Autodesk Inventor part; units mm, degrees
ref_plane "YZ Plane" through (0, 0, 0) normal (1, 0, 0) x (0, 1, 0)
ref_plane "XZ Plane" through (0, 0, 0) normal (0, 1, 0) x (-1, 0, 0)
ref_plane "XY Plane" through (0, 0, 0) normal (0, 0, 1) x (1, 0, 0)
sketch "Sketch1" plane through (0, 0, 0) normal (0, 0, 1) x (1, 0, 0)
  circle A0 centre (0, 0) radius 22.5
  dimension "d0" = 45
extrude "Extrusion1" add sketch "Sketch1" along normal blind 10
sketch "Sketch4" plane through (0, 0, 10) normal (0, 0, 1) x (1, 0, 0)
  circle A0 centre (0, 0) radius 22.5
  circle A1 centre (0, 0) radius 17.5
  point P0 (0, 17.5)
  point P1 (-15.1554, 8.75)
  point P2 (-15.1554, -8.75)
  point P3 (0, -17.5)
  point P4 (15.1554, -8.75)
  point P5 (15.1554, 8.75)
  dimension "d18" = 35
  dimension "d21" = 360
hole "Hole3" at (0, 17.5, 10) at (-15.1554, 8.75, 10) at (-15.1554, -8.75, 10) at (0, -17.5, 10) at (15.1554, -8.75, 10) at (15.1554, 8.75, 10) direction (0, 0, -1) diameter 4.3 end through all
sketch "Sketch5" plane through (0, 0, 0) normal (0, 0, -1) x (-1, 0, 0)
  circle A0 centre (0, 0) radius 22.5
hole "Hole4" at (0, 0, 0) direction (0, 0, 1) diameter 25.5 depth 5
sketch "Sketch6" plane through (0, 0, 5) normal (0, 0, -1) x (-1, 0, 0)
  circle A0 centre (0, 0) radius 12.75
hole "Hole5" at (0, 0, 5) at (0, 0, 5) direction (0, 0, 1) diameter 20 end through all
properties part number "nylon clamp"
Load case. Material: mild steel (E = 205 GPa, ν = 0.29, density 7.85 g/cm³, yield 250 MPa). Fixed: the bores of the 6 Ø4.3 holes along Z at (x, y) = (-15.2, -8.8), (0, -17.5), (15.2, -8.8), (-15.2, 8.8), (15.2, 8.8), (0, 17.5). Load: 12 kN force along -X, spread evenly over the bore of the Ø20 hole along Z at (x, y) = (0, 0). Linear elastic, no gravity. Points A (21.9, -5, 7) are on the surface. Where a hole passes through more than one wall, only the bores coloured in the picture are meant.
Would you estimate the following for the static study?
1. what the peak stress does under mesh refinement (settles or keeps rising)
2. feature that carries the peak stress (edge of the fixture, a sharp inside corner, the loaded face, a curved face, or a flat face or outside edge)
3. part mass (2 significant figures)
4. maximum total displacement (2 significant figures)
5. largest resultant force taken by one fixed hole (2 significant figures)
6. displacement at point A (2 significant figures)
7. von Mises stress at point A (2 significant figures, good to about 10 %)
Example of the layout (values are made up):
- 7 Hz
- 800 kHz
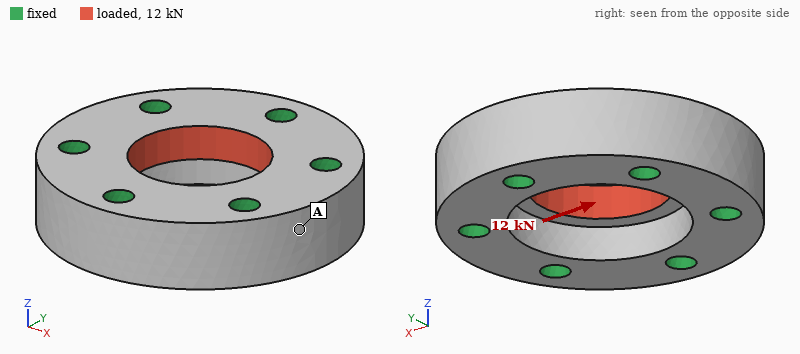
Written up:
- keeps rising
- edge of the fixture
- 86 g
- 2.3 µm
- 2.4 kN
- 0.61 µm
- 11 MPa
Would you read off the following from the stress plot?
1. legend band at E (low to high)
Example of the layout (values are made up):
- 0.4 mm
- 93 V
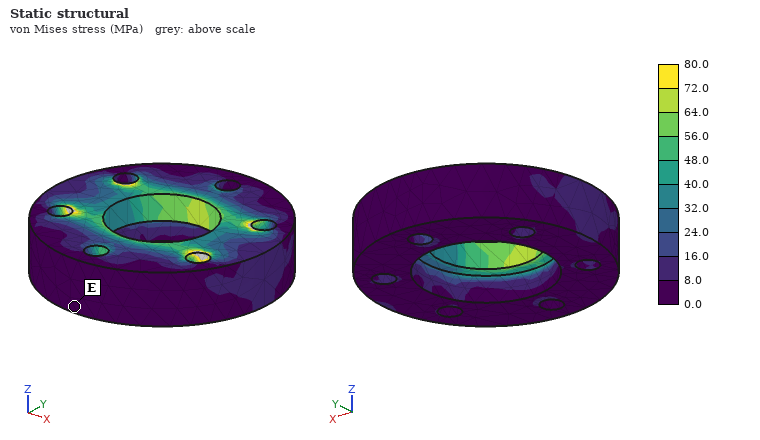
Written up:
- 0.0 to 8.0 MPa
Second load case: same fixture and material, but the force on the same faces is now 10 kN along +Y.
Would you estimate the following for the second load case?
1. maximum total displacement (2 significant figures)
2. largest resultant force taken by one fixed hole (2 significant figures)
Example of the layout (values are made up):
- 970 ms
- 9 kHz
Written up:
- 1.8 µm
- 2.2 kN
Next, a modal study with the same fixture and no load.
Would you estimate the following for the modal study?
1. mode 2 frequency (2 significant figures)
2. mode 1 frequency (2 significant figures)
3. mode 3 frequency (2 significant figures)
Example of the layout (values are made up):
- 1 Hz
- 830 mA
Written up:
- 75 kHz
- 74 kHz
- 76 kHz
